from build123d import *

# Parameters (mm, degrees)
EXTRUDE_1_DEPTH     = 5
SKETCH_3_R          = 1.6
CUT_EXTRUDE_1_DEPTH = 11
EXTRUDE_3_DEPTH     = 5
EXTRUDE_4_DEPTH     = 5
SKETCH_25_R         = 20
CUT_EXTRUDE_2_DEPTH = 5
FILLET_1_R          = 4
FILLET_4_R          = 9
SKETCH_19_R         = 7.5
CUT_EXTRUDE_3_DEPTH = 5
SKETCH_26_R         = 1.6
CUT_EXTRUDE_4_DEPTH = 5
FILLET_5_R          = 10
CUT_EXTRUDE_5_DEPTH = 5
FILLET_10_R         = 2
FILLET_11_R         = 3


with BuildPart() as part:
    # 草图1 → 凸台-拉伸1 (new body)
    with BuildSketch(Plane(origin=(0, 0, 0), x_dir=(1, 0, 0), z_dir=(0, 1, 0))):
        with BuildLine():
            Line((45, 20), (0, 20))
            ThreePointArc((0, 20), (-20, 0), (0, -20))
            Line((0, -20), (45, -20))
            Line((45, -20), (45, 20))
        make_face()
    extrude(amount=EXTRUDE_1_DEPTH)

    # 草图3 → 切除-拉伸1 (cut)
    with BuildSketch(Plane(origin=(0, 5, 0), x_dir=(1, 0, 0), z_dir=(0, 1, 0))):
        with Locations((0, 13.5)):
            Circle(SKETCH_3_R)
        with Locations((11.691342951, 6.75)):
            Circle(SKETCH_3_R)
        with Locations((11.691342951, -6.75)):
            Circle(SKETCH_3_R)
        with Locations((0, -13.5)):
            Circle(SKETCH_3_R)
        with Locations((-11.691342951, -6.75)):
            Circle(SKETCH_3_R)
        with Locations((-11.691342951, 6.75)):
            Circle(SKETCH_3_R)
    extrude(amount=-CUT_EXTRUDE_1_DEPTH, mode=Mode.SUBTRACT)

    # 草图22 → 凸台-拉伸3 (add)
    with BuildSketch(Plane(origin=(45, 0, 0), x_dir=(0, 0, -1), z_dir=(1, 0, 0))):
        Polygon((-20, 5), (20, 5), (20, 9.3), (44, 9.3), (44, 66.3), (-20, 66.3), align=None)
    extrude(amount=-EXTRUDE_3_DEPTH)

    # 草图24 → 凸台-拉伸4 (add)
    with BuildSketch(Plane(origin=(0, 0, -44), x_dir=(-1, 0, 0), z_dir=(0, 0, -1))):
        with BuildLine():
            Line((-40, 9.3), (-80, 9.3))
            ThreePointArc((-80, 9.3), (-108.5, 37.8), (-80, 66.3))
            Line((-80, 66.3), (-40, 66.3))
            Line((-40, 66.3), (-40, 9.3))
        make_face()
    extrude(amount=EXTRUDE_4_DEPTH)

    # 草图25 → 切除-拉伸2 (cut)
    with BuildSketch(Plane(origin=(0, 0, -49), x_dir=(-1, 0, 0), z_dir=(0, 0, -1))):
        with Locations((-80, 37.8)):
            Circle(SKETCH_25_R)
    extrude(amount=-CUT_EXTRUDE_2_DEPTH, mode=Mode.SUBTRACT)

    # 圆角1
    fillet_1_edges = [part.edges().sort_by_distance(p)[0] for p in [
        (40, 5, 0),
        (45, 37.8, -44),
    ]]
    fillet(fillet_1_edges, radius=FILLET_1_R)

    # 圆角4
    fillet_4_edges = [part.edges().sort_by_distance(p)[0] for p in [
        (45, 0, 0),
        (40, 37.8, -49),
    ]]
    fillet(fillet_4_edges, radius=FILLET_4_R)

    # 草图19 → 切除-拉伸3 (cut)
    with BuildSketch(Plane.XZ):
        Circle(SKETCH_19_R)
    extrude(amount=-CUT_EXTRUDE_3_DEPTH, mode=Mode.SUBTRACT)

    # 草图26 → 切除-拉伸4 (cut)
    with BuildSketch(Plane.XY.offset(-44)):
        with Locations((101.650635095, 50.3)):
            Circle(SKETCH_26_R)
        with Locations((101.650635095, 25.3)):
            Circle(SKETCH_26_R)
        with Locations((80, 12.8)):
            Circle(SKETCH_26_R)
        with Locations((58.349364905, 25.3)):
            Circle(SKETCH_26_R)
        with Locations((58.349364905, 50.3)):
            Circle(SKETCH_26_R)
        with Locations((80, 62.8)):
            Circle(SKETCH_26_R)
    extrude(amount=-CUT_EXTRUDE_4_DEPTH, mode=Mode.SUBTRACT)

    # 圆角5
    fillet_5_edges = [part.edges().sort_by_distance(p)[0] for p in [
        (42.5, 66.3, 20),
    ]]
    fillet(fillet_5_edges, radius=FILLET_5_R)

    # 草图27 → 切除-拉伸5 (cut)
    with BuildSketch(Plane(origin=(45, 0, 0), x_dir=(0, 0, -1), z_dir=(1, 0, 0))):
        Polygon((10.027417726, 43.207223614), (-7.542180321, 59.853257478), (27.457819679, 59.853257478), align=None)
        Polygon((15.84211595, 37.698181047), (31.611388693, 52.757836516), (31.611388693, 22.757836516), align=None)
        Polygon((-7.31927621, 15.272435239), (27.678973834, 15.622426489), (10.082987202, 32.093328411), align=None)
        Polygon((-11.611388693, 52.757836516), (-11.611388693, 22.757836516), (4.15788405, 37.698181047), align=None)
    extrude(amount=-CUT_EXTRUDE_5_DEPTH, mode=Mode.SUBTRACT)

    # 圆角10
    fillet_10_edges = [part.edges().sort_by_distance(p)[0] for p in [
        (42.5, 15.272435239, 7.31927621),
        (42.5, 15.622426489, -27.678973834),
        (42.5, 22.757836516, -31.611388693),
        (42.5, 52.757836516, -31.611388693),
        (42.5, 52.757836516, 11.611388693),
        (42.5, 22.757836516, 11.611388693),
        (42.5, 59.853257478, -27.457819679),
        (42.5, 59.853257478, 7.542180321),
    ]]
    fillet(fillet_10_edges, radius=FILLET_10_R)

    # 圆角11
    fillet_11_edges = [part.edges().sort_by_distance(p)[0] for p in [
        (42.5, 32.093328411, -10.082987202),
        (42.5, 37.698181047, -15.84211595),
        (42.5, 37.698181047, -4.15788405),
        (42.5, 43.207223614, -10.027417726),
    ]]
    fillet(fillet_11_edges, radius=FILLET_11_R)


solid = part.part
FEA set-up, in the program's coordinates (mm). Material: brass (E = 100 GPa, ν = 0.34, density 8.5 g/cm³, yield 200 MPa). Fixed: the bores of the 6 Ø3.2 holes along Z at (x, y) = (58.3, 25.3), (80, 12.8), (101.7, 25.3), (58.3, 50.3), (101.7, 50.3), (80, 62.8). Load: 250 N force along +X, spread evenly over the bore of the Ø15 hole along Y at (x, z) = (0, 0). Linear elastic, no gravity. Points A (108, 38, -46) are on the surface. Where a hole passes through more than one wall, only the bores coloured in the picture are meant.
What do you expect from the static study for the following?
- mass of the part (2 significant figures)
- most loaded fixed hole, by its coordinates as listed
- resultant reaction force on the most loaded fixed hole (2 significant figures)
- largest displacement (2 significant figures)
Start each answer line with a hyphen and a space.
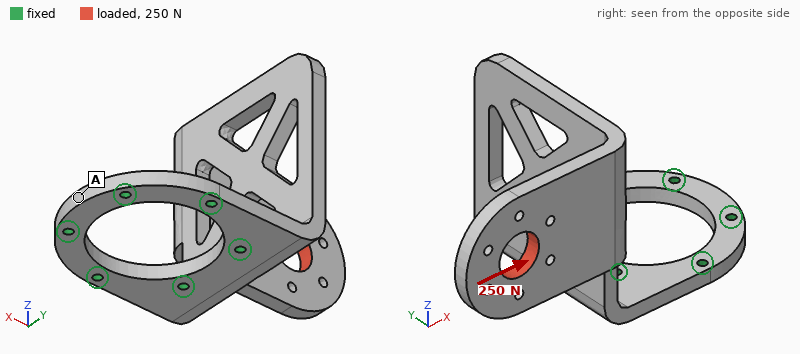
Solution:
- 300 g
- (58.3, 25.3)
- 280 N
- 1.2 mm
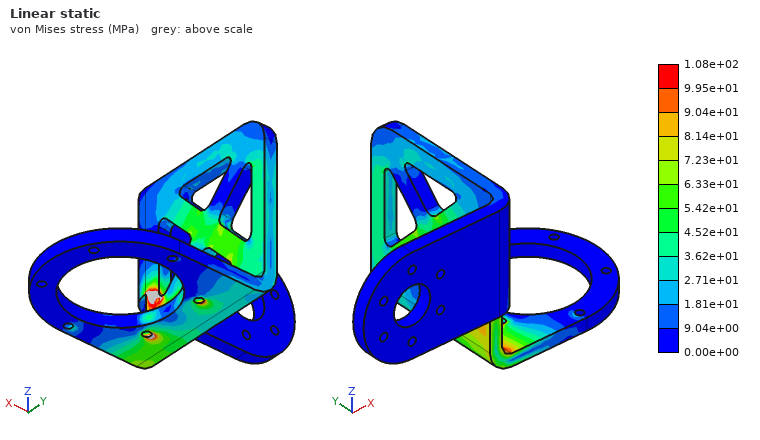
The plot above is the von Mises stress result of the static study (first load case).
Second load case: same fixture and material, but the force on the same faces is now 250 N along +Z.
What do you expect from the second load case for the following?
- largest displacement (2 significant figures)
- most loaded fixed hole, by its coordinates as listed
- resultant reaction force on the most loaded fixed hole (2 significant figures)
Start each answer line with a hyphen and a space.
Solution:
- 1.5 mm
- (58.3, 25.3)
- 540 N
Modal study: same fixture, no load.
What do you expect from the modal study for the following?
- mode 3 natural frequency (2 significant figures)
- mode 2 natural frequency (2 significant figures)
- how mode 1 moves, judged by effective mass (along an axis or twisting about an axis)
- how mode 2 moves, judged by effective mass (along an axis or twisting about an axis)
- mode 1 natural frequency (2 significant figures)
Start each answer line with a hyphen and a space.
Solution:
- 870 Hz
- 390 Hz
- along X
- along Y
- 230 Hz
